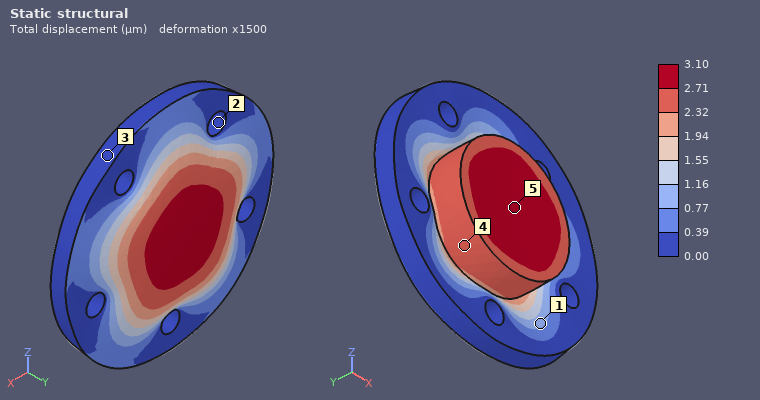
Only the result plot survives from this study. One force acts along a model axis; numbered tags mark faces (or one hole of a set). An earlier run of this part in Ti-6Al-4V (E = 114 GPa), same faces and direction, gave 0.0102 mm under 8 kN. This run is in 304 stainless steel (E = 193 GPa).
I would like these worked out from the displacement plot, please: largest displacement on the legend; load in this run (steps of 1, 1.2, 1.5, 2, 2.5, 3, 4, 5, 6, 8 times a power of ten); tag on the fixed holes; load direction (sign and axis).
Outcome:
3.10 µm
4 kN
2
+Y
